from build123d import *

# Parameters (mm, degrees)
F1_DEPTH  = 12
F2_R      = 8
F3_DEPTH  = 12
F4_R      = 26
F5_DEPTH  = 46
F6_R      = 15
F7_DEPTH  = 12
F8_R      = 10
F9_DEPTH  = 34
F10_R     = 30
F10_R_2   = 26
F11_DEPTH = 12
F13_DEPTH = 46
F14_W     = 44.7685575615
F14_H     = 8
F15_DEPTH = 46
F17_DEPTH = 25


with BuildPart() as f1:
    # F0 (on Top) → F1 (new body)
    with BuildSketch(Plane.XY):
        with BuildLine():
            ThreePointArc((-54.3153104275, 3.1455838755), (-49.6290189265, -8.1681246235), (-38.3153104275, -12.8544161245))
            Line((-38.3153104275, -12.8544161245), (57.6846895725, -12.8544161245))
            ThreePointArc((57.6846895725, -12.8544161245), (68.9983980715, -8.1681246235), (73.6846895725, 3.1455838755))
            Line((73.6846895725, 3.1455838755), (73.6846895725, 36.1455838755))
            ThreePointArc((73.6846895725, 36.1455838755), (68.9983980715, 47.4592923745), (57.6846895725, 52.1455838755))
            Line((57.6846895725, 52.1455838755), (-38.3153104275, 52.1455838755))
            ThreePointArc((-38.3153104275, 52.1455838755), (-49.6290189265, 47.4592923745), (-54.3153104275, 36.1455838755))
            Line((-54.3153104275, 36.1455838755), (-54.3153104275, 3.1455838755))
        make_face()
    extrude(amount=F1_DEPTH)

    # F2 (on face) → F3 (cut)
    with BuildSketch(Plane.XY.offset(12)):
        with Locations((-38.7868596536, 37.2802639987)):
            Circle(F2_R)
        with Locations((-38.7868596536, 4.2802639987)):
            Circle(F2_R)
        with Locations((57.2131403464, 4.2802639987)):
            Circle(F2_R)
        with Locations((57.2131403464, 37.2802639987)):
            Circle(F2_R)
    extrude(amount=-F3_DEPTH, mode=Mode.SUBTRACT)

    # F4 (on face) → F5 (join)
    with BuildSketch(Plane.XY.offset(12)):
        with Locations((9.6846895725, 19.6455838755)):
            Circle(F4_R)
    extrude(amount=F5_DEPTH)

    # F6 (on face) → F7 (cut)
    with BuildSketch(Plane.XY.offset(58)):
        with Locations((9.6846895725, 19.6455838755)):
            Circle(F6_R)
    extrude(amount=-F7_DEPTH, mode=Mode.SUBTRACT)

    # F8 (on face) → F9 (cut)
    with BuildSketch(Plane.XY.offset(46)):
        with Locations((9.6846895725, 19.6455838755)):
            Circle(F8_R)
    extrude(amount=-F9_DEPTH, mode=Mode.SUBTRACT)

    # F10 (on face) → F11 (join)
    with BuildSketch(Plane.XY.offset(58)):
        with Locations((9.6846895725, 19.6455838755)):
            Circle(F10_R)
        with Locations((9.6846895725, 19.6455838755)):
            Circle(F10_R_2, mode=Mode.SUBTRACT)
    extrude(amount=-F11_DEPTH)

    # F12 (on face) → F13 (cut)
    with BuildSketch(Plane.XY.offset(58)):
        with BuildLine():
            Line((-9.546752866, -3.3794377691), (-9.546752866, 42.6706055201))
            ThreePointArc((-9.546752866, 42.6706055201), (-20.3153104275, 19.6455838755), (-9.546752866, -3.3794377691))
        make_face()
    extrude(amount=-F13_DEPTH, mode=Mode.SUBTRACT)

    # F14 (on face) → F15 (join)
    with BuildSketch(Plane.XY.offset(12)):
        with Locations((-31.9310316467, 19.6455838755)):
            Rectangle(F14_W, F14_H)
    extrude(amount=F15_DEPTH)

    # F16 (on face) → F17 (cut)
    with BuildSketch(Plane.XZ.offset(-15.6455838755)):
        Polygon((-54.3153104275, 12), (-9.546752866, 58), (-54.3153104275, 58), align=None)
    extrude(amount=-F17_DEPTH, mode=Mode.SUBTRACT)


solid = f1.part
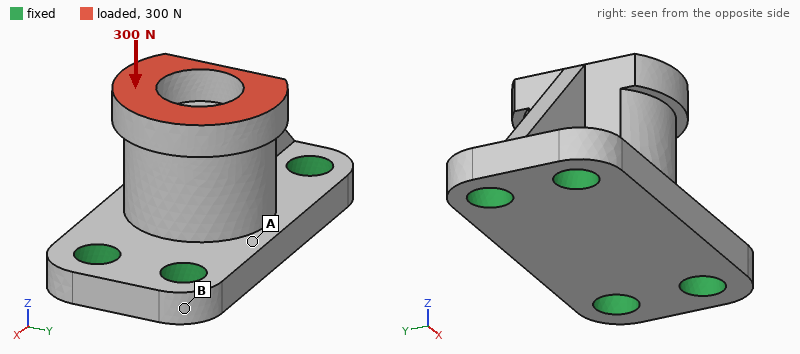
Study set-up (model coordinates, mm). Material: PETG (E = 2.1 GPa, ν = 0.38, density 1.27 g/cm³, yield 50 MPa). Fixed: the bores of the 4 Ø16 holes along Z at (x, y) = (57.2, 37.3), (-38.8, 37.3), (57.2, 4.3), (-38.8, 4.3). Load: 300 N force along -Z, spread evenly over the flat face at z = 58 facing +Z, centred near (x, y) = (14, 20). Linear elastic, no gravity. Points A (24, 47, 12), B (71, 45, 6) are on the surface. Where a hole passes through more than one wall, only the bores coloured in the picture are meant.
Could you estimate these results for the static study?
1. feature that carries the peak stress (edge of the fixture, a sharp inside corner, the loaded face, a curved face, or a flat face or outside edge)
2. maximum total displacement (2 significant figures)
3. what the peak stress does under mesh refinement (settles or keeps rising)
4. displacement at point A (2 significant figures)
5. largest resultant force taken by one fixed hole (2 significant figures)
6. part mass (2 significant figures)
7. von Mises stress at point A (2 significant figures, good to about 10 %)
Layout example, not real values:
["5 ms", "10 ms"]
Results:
["edge of the fixture", "30 µm", "keeps rising", "19 µm", "99 N", "220 g", "0.47 MPa"]
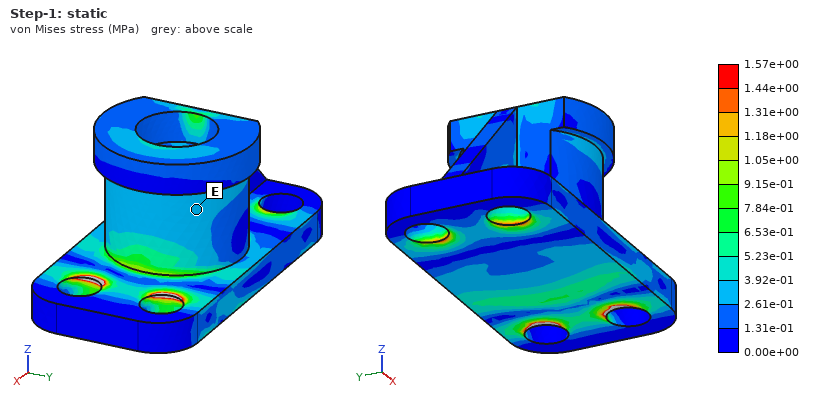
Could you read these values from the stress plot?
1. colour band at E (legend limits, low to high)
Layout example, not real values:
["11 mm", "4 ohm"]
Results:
["2.61e-01 to 3.92e-01 MPa"]
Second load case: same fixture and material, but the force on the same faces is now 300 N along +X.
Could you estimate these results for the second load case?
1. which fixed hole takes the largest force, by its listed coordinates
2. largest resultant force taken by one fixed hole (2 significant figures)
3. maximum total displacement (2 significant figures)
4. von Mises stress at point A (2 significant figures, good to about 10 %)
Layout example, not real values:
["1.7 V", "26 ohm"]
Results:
["(-38.8, 4.3)", "150 N", "73 µm", "0.60 MPa"]
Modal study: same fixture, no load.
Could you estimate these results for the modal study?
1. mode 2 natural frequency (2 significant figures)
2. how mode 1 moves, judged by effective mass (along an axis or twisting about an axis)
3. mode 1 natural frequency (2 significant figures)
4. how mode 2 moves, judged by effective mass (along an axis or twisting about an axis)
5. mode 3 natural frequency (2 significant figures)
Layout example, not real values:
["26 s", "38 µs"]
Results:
["1500 Hz", "along Y", "880 Hz", "along Z", "2000 Hz"]
